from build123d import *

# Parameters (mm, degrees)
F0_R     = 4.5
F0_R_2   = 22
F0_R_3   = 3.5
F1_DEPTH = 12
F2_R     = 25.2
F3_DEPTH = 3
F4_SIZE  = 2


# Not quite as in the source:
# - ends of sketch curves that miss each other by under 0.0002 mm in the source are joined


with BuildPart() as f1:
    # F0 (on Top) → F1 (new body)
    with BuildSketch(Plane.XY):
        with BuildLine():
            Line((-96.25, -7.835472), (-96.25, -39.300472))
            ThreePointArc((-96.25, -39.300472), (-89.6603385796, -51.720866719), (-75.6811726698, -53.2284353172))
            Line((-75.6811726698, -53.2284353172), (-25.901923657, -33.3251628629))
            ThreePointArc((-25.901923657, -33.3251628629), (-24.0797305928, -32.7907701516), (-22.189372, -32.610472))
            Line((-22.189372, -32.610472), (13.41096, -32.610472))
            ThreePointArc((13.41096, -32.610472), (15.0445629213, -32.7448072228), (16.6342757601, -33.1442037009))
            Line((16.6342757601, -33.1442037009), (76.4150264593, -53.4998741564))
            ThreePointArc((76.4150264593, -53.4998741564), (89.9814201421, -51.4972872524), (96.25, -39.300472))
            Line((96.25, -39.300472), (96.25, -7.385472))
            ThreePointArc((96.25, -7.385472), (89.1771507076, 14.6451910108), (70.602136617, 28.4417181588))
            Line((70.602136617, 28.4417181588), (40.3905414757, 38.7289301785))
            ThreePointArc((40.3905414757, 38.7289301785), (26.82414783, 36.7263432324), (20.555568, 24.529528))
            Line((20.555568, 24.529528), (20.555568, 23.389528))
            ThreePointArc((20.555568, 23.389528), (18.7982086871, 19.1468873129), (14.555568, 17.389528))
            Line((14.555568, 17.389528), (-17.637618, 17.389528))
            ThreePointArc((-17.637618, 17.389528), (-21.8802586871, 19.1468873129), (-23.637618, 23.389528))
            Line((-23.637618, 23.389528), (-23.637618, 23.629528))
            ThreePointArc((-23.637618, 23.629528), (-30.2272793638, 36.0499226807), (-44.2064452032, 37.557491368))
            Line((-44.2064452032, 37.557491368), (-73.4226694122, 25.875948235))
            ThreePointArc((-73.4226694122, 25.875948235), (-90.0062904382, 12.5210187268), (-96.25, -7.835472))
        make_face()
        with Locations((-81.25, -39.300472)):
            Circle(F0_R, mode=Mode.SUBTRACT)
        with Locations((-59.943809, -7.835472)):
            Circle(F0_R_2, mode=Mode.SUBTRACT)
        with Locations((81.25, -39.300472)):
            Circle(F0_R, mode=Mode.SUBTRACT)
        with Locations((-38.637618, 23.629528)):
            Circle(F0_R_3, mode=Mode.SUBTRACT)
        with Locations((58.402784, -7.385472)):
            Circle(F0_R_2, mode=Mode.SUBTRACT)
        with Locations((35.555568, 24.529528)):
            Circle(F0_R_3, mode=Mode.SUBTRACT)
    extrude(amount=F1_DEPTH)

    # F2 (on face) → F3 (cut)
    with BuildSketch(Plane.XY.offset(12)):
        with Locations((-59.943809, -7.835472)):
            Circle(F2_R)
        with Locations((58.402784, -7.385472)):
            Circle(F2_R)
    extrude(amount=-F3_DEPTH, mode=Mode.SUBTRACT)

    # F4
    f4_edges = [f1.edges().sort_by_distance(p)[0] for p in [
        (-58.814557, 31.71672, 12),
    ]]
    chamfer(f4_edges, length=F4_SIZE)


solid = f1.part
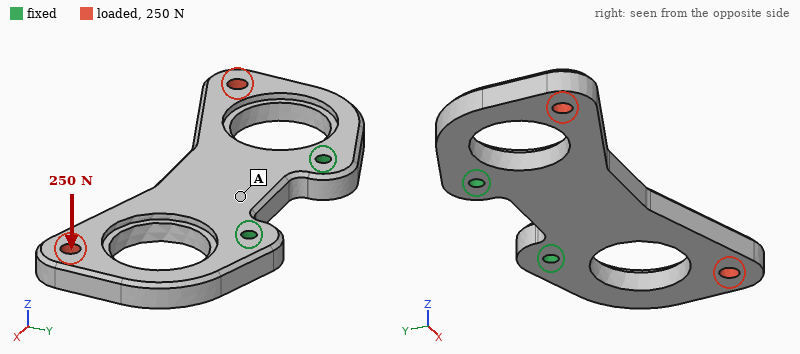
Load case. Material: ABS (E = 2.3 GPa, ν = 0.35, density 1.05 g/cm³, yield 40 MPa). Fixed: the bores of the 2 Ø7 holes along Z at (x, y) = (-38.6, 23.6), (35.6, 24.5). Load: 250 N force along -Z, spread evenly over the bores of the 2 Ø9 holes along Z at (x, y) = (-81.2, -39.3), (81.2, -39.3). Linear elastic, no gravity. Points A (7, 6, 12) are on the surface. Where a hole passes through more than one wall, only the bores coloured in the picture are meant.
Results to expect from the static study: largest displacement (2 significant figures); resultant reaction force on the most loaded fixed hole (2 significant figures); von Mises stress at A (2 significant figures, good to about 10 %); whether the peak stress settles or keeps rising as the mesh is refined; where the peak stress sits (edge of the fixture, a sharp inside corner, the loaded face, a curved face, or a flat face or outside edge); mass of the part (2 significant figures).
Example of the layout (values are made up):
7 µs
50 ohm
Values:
2.5 mm
130 N
2.0 MPa
keeps rising
edge of the fixture
120 g
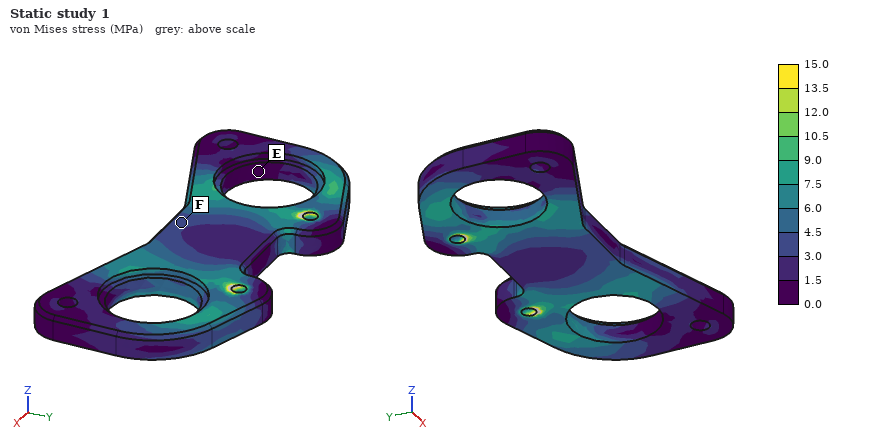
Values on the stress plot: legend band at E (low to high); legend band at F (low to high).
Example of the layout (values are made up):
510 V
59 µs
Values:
0.0 to 1.5 MPa
3.0 to 4.5 MPa
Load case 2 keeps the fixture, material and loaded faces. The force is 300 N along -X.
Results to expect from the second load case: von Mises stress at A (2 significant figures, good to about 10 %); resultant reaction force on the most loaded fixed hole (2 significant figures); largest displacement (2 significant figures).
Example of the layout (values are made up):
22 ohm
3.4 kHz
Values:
0.65 MPa
280 N
0.11 mm
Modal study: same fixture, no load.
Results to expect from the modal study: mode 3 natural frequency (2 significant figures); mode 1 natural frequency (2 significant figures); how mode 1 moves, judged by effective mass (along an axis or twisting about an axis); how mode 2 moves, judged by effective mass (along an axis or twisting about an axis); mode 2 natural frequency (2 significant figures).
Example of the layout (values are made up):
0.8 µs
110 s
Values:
680 Hz
320 Hz
along Z
twisting about Y
360 Hz
